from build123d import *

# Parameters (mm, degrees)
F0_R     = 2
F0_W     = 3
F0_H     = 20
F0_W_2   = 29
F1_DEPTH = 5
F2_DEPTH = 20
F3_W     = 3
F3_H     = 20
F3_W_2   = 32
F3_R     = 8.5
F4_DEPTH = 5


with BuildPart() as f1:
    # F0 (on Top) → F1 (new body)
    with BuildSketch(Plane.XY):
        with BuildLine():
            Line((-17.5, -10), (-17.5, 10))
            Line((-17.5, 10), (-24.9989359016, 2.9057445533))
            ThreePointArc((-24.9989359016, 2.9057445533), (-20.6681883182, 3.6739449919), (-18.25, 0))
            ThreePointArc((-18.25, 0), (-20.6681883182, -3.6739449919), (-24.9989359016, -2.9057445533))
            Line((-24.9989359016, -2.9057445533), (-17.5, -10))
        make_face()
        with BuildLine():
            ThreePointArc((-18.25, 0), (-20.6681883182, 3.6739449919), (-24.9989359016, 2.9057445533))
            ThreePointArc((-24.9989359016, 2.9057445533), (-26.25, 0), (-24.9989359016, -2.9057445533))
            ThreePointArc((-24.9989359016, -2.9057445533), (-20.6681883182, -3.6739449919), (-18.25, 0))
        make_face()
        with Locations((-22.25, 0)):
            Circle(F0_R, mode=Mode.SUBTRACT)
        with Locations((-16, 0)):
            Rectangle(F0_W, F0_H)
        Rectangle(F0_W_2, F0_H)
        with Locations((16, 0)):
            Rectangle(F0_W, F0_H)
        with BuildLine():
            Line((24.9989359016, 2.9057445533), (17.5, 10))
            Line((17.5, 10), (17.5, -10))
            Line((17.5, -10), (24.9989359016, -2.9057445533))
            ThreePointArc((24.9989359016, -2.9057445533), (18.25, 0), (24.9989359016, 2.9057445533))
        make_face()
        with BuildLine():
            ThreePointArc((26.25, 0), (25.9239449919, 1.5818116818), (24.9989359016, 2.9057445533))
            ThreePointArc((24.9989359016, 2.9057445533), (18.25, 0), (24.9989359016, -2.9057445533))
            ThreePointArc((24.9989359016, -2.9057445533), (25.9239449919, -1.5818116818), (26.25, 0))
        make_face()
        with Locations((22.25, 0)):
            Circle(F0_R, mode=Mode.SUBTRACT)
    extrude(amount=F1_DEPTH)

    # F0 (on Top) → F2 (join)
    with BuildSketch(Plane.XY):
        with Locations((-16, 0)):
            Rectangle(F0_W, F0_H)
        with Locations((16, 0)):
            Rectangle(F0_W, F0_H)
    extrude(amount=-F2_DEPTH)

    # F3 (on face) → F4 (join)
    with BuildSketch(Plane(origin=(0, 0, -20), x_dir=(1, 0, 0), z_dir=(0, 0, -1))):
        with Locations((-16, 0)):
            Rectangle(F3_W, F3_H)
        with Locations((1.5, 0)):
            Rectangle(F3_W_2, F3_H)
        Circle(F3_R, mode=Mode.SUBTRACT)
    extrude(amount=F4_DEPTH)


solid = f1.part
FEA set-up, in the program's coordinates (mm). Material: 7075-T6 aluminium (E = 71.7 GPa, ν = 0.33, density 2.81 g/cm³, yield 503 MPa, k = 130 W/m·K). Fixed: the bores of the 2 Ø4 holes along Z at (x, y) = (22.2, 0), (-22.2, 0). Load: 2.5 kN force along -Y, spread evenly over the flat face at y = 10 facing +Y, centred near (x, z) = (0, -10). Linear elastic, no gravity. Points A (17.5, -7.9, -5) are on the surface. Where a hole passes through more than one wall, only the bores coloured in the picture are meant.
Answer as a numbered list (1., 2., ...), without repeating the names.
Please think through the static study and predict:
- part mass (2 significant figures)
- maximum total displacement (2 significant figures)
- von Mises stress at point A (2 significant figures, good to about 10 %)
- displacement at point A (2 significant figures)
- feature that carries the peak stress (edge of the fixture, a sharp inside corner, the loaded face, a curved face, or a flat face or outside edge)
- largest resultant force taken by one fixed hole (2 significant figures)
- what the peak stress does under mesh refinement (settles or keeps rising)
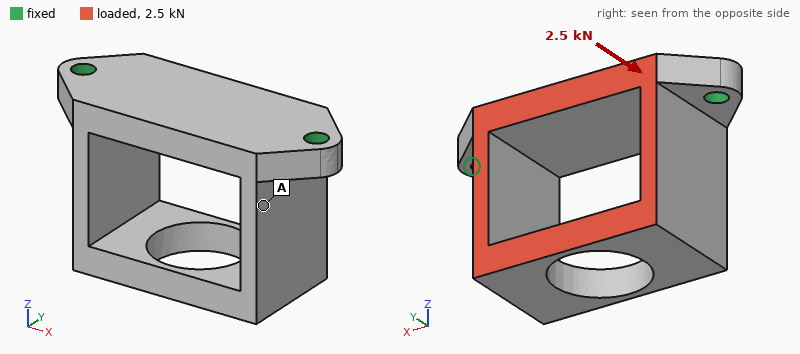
1. 26 g
2. 0.21 mm
3. 54 MPa
4. 0.070 mm
5. edge of the fixture
6. 1.3 kN
7. keeps rising
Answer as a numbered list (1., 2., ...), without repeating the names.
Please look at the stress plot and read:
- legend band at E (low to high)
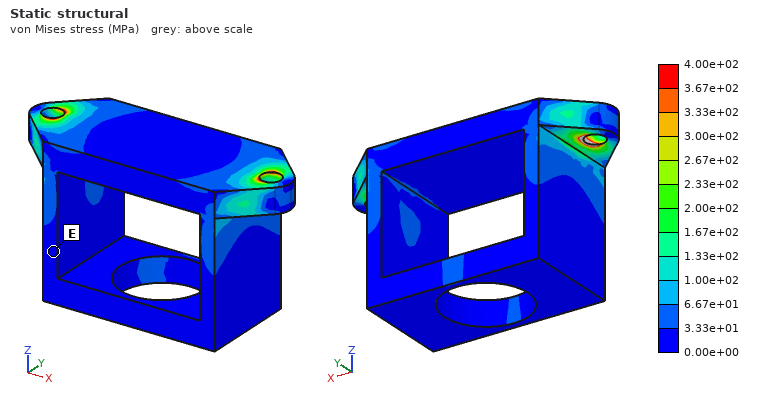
1. 0.00e+00 to 3.33e+01 MPa
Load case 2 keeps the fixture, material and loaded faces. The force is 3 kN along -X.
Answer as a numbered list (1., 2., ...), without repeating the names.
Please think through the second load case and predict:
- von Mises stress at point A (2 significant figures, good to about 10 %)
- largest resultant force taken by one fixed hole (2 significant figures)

1. 150 MPa
2. 1.8 kN
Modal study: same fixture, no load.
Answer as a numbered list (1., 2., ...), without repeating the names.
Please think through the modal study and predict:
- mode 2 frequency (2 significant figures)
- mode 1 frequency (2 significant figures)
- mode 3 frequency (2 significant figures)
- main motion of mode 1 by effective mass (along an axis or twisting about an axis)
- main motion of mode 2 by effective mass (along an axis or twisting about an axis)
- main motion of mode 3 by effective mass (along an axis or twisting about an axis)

1. 4400 Hz
2. 3900 Hz
3. 7100 Hz
4. along X
5. along Y
6. twisting about Z
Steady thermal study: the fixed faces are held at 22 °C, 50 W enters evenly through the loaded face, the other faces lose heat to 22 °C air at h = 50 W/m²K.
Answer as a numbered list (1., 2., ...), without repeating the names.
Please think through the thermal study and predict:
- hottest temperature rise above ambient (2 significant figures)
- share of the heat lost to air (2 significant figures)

1. 63 K
2. 14 %
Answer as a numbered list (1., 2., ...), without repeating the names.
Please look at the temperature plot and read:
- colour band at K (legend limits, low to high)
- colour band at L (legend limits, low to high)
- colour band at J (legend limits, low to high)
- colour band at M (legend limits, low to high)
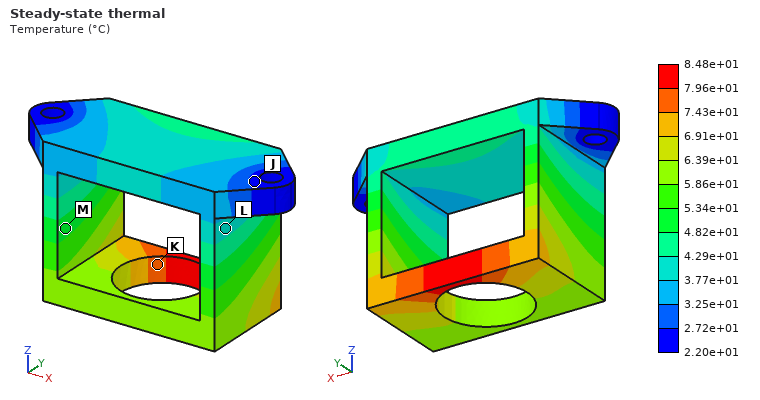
1. 7.43e+01 to 7.96e+01 °C
2. 3.77e+01 to 4.29e+01 °C
3. 2.20e+01 to 2.72e+01 °C
4. 4.82e+01 to 5.34e+01 °C
